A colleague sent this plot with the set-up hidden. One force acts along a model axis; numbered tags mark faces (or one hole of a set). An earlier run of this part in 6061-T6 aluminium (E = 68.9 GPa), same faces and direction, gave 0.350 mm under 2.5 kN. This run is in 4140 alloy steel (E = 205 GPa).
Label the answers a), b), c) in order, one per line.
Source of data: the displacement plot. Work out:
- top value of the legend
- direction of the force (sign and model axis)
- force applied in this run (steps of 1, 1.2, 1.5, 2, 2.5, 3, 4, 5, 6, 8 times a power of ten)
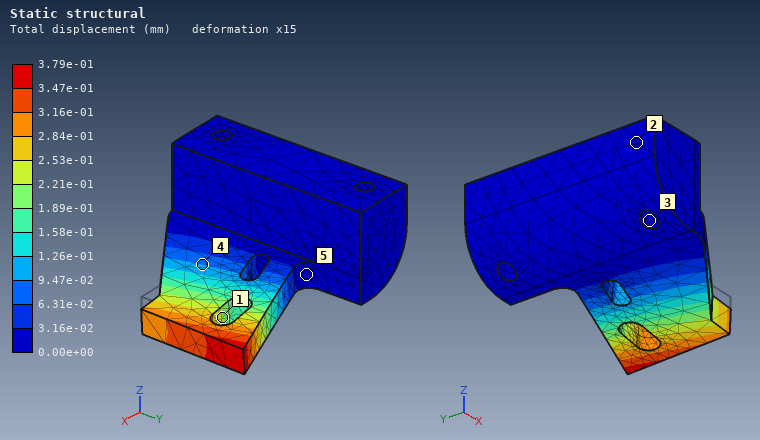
a) 3.79e-01 mm
b) -Z
c) 8 kN
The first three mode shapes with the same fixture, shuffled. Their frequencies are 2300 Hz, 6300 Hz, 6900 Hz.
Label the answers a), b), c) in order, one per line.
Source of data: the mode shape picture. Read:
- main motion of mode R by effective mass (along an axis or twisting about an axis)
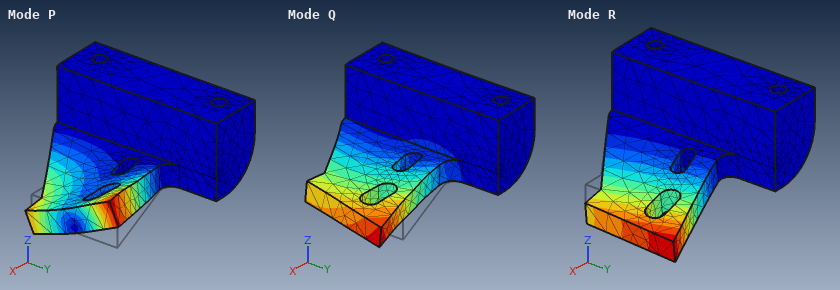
a) along Z
